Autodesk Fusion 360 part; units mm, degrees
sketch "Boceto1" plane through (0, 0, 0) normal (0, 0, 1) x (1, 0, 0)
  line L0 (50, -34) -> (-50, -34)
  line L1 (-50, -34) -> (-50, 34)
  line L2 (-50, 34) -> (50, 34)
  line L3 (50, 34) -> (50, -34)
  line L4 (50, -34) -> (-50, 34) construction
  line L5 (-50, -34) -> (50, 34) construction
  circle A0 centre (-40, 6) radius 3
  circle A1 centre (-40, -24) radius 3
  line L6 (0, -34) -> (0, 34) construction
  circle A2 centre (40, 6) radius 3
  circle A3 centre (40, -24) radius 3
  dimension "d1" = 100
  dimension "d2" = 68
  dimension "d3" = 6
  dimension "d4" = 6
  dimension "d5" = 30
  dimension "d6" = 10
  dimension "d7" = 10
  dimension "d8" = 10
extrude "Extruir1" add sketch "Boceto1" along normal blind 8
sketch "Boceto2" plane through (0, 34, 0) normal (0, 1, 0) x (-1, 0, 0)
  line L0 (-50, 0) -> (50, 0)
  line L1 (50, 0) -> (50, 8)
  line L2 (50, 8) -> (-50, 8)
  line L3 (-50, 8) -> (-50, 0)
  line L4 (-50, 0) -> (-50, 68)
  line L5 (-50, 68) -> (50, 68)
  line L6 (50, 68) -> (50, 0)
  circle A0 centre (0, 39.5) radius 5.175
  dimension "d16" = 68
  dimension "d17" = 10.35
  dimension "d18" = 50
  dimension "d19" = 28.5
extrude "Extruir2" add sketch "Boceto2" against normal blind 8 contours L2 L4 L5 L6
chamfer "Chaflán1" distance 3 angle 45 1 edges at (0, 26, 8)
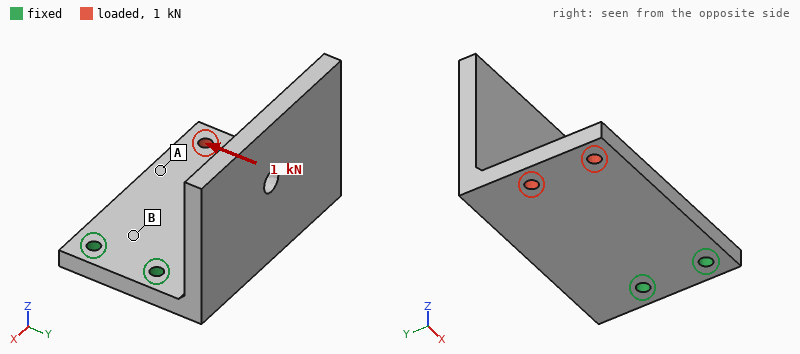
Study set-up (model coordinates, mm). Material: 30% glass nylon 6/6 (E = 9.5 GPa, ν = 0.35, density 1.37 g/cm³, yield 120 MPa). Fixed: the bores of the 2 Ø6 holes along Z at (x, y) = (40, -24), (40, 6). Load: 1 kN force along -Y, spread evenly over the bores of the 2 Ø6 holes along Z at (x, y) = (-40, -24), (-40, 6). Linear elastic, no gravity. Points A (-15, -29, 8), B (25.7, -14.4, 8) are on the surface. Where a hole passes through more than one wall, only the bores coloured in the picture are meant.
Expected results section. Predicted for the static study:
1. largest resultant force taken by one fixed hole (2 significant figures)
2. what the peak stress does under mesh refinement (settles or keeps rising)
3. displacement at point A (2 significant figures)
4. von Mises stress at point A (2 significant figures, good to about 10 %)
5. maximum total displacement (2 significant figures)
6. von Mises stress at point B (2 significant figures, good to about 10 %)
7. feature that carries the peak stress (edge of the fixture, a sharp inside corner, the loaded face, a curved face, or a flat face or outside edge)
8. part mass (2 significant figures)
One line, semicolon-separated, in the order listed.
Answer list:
2.4 kN; keeps rising; 0.17 mm; 4.0 MPa; 0.29 mm; 11 MPa; edge of the fixture; 140 g
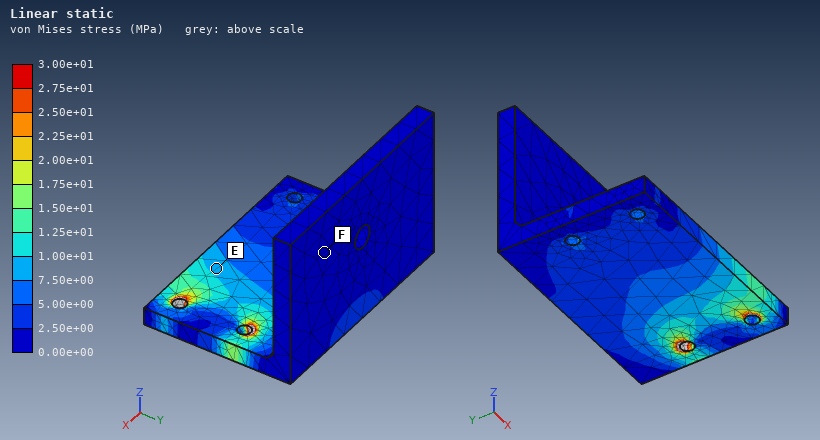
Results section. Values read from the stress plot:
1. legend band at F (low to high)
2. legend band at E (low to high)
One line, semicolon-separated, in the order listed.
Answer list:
0.00e+00 to 2.50e+00 MPa; 7.50e+00 to 1.00e+01 MPa
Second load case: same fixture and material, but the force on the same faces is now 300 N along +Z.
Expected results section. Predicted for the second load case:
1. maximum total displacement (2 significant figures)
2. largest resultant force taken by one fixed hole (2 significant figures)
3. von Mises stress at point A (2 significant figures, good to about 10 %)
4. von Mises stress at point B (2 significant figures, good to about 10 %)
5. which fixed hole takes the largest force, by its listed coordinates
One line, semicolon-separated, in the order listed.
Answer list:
1.6 mm; 190 N; 7.2 MPa; 19 MPa; (40, 6)
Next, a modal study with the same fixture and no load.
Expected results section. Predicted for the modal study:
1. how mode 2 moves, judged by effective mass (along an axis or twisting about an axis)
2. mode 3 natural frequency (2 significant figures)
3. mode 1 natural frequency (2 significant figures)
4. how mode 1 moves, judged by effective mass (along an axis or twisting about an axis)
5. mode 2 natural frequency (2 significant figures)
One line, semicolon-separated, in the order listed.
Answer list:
along Y; 1100 Hz; 290 Hz; along Z; 450 Hz
